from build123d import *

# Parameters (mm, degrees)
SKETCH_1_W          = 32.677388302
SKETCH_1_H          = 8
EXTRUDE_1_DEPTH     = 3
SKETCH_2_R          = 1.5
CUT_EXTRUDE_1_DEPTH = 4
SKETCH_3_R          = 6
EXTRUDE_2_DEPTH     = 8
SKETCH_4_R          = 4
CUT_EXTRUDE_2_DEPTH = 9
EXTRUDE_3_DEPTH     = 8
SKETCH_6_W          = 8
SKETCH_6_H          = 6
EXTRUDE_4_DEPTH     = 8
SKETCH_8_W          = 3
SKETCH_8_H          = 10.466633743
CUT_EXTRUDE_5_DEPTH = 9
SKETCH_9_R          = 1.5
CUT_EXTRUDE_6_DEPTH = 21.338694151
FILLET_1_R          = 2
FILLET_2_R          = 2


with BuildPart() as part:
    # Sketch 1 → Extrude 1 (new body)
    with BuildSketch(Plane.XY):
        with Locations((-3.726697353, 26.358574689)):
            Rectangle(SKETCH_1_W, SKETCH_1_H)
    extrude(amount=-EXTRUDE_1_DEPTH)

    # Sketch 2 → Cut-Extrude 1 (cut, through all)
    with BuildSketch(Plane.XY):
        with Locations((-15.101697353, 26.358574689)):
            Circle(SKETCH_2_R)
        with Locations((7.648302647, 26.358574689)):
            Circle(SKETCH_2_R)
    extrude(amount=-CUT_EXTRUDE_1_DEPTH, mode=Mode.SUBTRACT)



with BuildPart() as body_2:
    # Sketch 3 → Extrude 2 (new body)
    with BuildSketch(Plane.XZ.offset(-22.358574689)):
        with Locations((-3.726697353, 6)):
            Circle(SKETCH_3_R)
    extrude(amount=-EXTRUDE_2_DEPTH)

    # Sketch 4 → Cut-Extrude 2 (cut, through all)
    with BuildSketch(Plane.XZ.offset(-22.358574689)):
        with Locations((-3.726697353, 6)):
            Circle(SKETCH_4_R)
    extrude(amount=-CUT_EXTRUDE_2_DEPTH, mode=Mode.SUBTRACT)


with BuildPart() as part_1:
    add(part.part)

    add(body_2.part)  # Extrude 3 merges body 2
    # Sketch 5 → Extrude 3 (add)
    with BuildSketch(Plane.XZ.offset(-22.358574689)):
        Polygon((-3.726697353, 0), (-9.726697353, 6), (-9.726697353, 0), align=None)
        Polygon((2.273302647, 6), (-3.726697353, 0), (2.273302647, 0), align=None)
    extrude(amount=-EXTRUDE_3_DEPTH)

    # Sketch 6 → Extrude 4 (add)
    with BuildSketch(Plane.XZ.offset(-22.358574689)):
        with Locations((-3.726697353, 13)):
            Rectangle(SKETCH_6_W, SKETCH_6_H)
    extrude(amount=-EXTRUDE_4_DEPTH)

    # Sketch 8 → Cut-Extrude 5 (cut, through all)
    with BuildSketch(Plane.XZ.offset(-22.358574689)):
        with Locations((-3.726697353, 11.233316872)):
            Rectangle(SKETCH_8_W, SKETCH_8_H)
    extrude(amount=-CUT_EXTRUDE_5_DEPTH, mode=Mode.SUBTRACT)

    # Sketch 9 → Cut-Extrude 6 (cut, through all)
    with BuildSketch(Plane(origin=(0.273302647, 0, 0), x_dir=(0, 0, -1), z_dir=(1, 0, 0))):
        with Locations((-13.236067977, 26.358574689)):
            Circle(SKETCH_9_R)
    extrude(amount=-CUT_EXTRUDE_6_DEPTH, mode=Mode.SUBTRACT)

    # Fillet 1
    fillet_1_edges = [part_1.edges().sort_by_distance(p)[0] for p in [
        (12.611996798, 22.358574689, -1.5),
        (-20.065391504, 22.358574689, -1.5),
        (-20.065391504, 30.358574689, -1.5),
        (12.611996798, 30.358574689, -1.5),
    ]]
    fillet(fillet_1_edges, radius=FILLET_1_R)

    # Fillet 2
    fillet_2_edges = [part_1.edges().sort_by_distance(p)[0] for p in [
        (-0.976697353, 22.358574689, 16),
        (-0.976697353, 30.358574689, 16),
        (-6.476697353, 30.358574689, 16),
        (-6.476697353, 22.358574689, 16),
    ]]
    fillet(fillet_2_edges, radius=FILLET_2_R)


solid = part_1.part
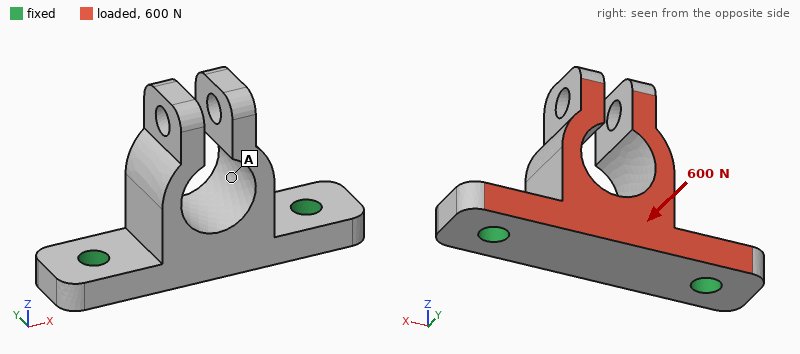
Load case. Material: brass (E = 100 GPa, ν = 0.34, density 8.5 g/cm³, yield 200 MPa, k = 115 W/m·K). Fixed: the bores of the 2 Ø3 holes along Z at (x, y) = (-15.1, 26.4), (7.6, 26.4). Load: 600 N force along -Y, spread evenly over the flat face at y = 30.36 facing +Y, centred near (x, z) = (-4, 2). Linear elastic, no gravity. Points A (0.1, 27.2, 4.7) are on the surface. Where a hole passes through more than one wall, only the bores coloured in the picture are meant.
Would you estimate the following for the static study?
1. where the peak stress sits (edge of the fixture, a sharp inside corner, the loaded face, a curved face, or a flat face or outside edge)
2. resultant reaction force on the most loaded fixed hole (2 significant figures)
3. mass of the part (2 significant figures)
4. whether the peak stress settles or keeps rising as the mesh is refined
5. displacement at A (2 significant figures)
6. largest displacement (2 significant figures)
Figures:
edge of the fixture
300 N
12 g
keeps rising
19 µm
52 µm
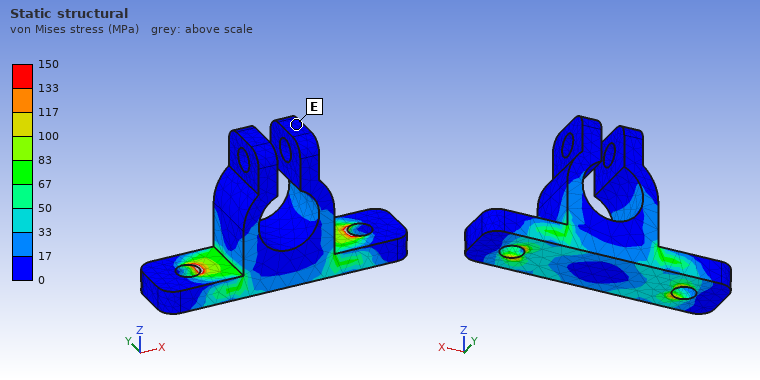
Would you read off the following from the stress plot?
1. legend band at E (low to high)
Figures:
0 to 17 MPa
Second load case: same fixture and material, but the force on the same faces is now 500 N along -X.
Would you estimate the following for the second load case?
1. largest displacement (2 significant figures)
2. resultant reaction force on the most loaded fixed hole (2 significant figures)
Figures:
39 µm
290 N
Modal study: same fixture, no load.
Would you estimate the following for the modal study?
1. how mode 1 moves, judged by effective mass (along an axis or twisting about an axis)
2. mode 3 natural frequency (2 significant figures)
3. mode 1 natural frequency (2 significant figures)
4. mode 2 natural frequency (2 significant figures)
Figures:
along Y
6200 Hz
5900 Hz
6200 Hz
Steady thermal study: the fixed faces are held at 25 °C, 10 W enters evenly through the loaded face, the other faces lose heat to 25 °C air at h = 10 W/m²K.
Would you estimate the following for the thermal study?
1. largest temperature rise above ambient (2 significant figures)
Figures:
16 K
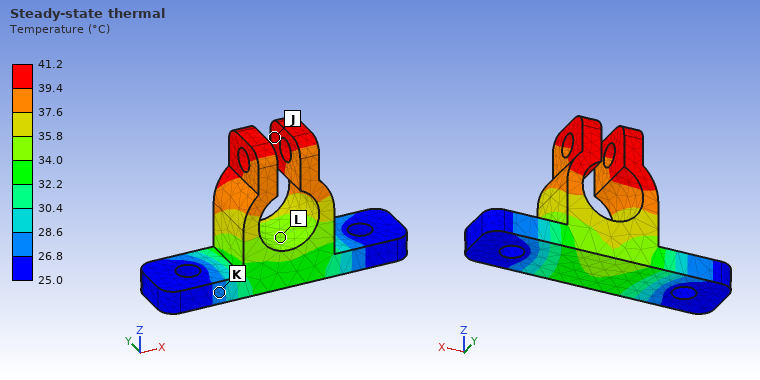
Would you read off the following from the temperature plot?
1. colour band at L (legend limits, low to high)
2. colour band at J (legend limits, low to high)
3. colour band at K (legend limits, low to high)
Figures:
34.0 to 35.8 °C
39.4 to 41.2 °C
26.8 to 28.6 °C
